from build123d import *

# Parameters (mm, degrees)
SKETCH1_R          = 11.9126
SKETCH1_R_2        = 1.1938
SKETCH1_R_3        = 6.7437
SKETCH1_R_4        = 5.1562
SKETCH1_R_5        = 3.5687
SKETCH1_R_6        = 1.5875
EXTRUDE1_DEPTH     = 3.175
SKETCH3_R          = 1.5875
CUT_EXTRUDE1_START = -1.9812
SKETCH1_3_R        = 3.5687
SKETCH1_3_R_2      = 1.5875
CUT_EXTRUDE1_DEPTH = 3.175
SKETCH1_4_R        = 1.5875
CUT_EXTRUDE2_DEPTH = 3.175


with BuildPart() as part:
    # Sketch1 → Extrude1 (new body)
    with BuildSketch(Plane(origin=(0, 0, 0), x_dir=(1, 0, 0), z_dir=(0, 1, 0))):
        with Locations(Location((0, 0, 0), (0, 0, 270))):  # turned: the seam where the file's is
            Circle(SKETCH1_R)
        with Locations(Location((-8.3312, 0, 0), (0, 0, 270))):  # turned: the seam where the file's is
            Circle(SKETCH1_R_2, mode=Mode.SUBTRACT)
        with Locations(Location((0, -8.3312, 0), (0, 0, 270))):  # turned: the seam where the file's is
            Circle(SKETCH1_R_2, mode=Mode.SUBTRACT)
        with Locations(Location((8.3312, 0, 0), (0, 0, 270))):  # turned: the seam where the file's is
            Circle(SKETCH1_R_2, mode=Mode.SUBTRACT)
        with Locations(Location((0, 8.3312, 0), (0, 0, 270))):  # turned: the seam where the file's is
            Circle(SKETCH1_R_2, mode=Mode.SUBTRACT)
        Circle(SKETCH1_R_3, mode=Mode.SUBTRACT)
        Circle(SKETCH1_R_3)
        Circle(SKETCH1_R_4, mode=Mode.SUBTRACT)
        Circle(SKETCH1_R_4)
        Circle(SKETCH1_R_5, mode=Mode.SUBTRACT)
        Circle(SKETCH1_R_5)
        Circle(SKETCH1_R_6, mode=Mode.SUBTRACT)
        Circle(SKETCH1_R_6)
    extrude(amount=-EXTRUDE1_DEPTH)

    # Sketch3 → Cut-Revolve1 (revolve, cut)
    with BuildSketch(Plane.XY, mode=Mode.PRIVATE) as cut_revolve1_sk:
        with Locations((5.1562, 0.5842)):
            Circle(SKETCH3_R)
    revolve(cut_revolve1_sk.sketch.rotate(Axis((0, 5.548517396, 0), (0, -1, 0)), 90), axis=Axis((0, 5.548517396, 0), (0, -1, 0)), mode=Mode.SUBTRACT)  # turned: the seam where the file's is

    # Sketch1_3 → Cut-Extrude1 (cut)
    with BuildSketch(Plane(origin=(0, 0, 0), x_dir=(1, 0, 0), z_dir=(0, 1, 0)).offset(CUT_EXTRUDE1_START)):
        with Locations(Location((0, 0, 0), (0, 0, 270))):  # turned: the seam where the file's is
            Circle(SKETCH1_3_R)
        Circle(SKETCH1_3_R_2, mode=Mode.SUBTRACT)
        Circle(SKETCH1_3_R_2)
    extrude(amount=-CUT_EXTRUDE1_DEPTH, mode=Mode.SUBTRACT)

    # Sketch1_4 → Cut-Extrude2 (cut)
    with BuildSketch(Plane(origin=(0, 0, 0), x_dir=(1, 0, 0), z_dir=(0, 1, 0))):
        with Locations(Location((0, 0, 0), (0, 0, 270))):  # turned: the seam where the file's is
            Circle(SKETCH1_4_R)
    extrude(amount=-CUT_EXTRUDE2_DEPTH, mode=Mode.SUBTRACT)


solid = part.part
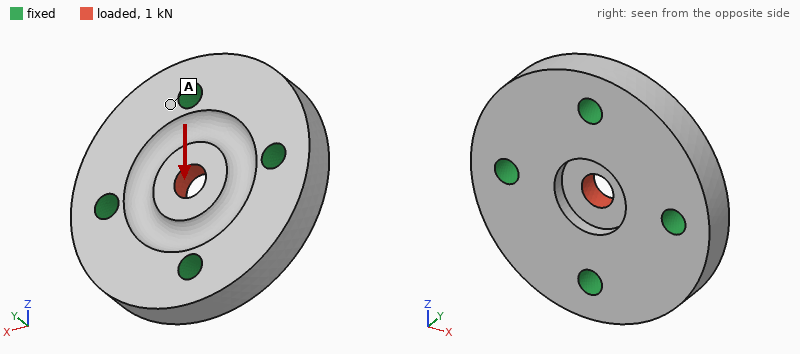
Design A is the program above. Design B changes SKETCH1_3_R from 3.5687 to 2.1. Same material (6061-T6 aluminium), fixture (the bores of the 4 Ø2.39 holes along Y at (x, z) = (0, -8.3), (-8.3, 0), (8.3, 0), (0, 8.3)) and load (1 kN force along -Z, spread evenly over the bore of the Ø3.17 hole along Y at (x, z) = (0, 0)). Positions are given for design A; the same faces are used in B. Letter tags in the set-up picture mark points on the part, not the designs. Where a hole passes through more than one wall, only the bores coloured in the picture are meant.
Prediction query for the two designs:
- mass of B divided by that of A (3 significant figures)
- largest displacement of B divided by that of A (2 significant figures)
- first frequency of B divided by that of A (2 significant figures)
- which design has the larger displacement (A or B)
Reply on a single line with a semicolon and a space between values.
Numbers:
1.03; 0.92; 1.0; A
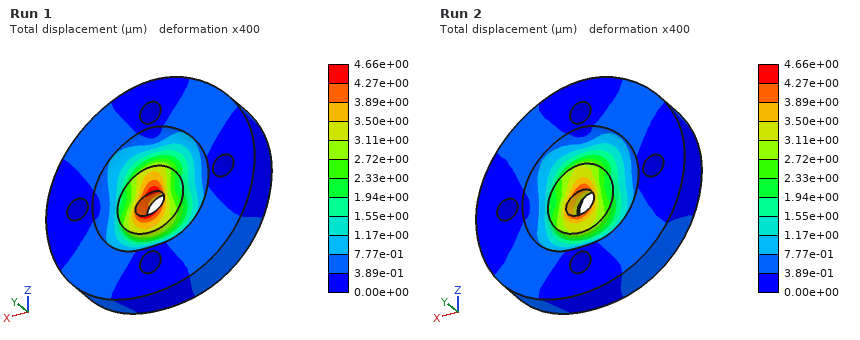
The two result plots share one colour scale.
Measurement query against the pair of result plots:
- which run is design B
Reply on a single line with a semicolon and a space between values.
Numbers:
Run 2
